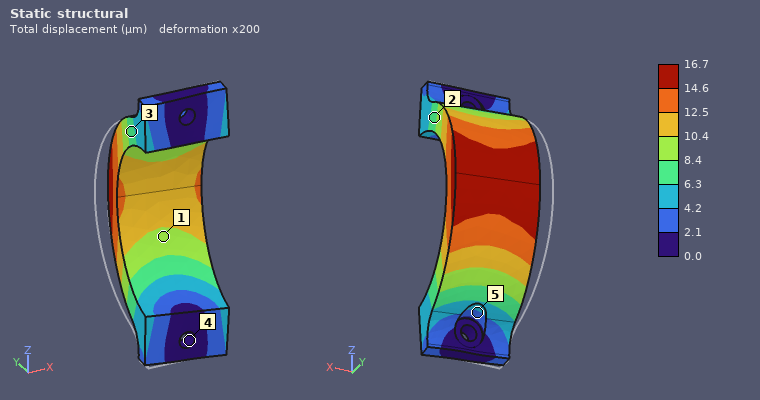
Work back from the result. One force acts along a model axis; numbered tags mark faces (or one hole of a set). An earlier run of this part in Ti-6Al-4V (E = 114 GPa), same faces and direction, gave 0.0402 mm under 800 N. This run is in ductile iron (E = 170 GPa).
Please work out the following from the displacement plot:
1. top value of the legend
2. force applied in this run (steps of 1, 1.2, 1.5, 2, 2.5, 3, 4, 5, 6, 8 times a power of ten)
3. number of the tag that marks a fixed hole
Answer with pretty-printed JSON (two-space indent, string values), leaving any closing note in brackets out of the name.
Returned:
{
  "top value of the legend": "16.7 µm",
  "force applied in this run": "500 N",
  "number of the tag that marks a fixed hole": "4"
}
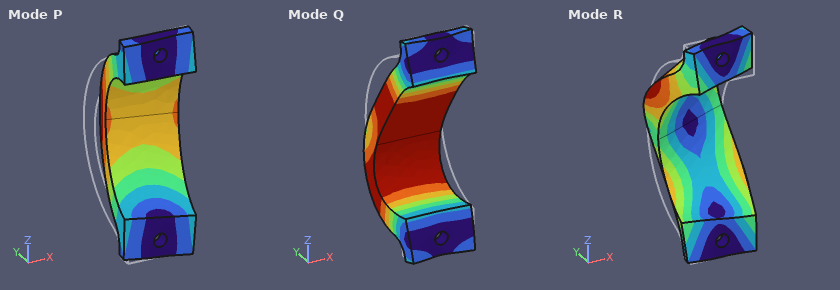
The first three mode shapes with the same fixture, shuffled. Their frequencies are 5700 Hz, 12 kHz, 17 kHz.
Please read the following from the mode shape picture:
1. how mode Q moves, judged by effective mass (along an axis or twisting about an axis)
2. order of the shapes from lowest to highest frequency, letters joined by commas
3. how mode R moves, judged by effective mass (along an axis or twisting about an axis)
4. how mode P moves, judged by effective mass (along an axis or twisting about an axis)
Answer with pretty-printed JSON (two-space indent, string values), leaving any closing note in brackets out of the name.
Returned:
{
  "how mode Q moves, judged by effective mass": "along Z",
  "order of the shapes from lowest to highest frequency, letters joined by commas": "P, Q, R",
  "how mode R moves, judged by effective mass": "twisting about Y",
  "how mode P moves, judged by effective mass": "along X"
}
